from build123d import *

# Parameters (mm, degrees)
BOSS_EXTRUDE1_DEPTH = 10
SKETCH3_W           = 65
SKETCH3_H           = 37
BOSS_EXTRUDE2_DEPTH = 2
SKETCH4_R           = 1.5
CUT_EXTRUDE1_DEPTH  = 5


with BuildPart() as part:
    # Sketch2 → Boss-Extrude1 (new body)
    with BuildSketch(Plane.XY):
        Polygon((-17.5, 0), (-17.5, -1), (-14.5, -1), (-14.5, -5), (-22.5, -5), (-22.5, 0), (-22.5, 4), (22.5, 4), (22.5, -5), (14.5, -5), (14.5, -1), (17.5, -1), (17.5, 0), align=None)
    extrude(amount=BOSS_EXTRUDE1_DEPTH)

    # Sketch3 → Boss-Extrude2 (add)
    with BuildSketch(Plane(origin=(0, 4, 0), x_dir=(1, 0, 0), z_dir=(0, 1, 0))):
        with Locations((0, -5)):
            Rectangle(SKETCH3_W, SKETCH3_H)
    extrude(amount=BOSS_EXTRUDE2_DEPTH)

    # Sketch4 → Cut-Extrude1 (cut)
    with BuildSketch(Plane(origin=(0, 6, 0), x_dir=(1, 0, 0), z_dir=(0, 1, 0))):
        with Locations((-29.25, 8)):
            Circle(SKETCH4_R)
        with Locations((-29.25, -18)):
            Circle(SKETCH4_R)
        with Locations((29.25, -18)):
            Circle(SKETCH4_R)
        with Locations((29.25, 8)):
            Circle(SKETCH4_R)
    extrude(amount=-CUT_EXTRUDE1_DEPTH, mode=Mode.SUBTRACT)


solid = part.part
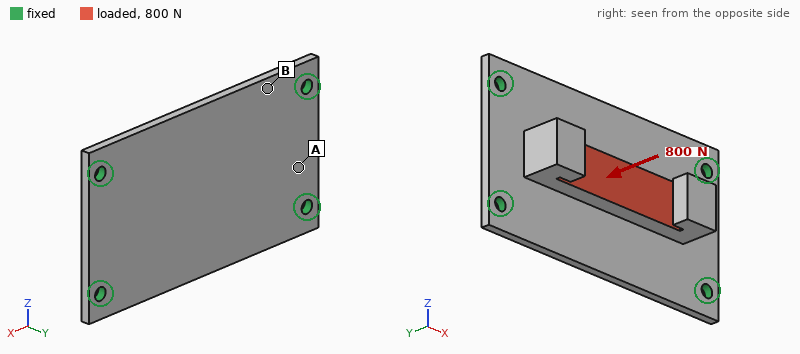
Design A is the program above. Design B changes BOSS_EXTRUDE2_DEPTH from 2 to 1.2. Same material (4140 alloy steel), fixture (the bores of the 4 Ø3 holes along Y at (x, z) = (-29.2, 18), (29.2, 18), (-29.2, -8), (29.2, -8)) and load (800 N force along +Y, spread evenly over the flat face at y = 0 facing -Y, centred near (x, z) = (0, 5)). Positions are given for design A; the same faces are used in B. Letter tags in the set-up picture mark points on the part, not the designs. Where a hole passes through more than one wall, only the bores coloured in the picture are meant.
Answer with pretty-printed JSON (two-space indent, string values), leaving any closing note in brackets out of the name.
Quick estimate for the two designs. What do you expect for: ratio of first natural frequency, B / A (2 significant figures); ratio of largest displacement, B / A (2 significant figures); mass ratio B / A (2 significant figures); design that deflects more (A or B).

{
  "ratio of first natural frequency, B / A": "0.68",
  "ratio of largest displacement, B / A": "2.5",
  "mass ratio B / A": "0.74",
  "design that deflects more": "B"
}
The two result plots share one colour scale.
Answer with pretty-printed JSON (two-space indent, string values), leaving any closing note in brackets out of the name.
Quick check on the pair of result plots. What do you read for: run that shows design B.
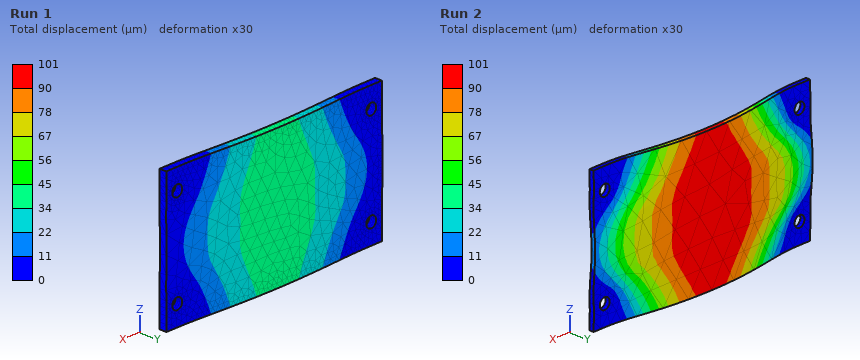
{
  "run that shows design B": "Run 2"
}
